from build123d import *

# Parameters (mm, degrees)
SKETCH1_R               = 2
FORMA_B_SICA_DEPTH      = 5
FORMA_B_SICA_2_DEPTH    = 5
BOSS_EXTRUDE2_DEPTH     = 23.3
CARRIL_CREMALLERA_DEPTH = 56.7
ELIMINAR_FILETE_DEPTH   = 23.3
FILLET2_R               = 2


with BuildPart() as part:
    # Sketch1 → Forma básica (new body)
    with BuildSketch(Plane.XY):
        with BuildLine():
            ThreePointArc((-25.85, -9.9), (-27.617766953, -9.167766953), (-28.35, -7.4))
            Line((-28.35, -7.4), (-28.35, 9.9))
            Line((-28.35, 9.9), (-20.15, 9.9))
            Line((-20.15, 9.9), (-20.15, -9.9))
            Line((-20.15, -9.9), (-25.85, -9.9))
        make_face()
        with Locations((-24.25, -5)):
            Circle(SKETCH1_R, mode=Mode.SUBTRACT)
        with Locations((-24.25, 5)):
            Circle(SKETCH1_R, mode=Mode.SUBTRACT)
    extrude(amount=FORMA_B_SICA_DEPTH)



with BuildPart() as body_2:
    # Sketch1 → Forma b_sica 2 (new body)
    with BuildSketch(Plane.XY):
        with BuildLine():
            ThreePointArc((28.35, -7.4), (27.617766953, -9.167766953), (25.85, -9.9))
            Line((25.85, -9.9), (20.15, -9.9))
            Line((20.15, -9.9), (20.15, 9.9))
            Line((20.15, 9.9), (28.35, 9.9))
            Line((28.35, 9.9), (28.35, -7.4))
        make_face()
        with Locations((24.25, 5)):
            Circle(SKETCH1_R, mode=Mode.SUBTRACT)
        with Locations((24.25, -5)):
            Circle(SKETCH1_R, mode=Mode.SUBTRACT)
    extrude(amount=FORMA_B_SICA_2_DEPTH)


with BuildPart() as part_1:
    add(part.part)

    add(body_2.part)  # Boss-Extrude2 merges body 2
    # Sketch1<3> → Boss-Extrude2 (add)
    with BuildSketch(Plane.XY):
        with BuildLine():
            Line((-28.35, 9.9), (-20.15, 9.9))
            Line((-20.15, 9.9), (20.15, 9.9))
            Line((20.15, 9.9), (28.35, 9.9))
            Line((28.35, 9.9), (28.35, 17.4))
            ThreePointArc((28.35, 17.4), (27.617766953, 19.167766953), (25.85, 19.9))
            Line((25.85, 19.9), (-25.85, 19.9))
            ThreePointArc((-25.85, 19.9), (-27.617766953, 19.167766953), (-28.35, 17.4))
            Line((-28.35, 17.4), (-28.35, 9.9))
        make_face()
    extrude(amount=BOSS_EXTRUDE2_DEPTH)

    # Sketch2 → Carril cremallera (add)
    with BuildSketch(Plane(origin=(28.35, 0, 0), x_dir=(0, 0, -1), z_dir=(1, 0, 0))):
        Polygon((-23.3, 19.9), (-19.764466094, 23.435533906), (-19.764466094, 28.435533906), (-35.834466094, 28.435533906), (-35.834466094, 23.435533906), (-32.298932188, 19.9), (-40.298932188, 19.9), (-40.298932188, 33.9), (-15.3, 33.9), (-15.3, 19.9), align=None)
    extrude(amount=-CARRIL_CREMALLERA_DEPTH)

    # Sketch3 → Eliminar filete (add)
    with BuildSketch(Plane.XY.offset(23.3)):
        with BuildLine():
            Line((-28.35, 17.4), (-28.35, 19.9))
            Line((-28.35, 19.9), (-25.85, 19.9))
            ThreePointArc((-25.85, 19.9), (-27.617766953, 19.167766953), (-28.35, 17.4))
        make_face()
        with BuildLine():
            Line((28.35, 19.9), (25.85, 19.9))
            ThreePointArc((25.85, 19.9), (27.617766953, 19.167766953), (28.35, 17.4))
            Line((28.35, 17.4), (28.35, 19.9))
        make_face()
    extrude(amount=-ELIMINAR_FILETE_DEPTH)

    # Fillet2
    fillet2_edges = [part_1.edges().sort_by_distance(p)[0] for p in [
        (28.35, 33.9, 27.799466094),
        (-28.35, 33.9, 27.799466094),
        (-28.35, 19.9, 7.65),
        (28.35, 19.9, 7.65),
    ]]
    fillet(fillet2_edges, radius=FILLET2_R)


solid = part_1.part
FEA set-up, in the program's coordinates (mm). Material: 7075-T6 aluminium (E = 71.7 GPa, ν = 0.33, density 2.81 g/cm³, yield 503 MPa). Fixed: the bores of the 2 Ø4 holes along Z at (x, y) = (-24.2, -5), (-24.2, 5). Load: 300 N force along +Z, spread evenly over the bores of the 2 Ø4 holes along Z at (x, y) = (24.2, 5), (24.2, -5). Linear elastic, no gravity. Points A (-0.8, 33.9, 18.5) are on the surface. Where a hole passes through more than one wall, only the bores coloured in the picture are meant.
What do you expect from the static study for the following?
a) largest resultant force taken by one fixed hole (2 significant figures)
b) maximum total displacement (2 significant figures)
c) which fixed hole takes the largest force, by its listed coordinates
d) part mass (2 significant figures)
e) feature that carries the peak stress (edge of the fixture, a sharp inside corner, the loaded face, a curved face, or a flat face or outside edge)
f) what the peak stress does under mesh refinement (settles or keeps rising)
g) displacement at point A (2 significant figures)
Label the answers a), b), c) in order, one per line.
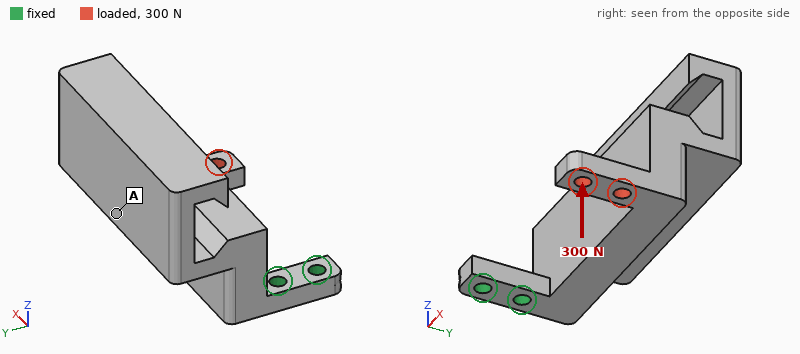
a) 290 N
b) 0.84 mm
c) (-24.2, 5)
d) 77 g
e) edge of the fixture
f) keeps rising
g) 0.28 mm
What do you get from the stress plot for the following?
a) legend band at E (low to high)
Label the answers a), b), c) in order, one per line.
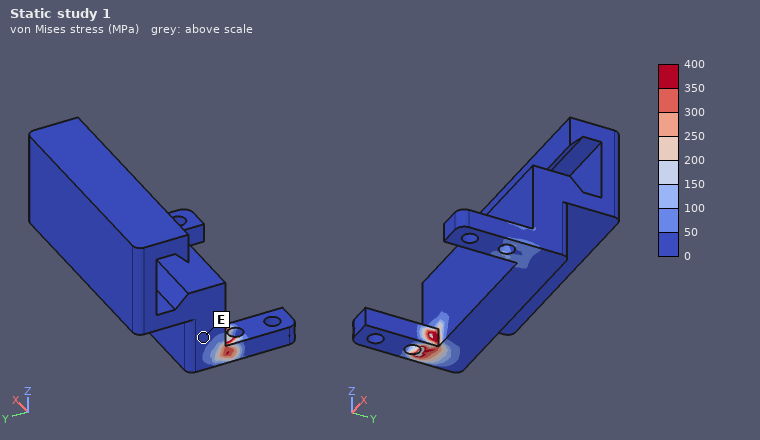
a) 0 to 50 MPa
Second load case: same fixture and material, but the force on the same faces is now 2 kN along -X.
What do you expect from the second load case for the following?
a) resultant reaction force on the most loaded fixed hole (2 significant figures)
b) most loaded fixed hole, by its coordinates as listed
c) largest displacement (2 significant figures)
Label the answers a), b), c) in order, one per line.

a) 1.7 kN
b) (-24.2, 5)
c) 0.93 mm
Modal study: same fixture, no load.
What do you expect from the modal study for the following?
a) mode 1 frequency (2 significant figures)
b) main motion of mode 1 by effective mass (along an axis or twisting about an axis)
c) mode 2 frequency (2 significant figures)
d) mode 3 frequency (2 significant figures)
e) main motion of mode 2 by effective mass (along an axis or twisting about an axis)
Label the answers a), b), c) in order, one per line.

a) 520 Hz
b) along Z
c) 600 Hz
d) 1200 Hz
e) along Y
